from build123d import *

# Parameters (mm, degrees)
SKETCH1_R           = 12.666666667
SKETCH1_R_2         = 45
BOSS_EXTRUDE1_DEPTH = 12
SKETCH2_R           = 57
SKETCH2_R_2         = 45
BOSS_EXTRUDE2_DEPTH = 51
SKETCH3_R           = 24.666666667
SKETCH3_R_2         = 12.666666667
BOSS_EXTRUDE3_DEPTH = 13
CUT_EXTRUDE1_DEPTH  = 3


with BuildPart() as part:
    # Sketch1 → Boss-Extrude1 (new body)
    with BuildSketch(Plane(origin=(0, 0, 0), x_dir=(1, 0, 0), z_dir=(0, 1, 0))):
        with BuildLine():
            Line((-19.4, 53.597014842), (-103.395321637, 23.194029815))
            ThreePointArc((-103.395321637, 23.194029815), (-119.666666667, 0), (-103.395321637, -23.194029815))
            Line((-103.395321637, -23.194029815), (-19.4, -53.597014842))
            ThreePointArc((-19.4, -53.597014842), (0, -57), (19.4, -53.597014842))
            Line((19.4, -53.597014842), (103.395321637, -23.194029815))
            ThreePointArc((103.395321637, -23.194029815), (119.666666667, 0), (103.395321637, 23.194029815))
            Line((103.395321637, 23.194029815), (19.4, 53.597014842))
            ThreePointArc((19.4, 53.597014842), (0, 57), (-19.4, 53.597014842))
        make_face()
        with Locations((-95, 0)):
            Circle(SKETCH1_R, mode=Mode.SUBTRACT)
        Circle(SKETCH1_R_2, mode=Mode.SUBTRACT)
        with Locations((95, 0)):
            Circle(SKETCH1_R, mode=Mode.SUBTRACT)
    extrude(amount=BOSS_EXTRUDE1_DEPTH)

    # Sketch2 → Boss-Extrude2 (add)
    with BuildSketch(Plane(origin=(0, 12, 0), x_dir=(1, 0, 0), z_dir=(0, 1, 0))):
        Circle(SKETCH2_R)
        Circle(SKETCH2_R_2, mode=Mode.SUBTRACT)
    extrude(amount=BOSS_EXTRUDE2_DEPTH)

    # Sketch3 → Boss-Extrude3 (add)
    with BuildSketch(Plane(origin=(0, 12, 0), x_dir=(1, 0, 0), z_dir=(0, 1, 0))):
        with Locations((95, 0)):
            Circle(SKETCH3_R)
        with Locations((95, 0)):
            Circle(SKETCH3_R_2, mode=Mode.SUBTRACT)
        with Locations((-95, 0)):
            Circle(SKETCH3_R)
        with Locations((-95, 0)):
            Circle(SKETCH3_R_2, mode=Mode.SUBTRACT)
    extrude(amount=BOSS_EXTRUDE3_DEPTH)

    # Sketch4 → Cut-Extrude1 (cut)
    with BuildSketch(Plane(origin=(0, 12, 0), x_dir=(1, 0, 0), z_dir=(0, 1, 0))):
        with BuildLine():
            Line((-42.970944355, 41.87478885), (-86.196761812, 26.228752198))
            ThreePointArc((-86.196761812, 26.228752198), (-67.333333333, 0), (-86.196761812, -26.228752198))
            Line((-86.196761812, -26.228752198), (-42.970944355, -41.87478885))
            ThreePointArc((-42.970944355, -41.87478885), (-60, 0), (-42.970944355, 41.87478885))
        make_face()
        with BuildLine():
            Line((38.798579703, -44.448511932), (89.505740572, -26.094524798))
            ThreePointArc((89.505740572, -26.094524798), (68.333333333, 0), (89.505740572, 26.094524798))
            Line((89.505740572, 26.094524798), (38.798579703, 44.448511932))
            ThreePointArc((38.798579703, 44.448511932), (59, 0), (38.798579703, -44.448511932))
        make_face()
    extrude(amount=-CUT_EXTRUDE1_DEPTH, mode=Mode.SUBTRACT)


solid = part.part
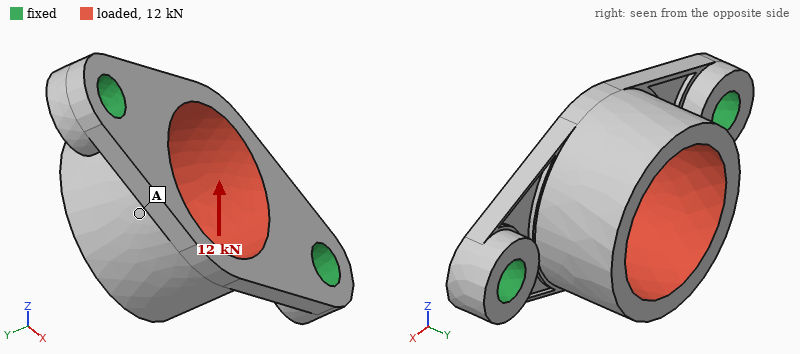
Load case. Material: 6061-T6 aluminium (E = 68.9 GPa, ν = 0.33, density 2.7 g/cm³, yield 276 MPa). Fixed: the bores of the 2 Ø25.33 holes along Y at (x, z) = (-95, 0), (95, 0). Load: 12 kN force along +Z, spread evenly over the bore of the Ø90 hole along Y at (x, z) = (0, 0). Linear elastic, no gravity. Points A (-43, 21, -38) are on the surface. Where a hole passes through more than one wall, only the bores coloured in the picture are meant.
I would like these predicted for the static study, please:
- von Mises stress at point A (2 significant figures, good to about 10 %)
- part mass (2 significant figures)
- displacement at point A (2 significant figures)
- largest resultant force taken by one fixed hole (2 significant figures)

15 MPa
960 g
0.18 mm
6.0 kN
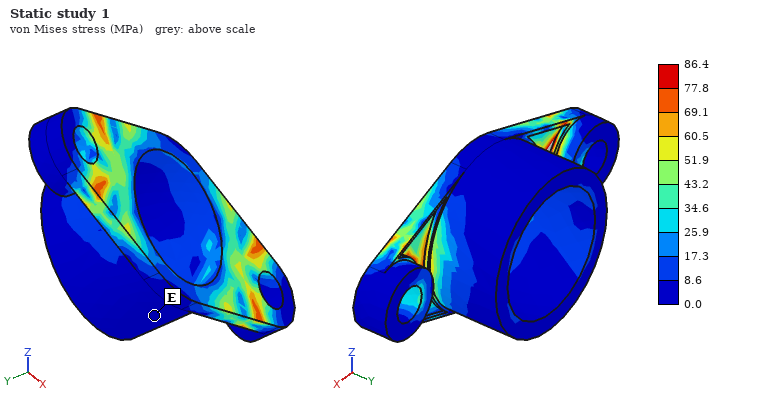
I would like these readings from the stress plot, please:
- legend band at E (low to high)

0.0 to 8.6 MPa
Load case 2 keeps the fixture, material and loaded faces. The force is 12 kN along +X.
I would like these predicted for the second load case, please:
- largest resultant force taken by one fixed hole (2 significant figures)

6.5 kN
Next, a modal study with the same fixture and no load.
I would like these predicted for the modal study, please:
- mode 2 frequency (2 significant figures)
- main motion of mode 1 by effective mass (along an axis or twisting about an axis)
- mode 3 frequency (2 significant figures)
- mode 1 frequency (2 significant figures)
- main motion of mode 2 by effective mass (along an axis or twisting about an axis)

2200 Hz
along Z
3700 Hz
1100 Hz
along Y
